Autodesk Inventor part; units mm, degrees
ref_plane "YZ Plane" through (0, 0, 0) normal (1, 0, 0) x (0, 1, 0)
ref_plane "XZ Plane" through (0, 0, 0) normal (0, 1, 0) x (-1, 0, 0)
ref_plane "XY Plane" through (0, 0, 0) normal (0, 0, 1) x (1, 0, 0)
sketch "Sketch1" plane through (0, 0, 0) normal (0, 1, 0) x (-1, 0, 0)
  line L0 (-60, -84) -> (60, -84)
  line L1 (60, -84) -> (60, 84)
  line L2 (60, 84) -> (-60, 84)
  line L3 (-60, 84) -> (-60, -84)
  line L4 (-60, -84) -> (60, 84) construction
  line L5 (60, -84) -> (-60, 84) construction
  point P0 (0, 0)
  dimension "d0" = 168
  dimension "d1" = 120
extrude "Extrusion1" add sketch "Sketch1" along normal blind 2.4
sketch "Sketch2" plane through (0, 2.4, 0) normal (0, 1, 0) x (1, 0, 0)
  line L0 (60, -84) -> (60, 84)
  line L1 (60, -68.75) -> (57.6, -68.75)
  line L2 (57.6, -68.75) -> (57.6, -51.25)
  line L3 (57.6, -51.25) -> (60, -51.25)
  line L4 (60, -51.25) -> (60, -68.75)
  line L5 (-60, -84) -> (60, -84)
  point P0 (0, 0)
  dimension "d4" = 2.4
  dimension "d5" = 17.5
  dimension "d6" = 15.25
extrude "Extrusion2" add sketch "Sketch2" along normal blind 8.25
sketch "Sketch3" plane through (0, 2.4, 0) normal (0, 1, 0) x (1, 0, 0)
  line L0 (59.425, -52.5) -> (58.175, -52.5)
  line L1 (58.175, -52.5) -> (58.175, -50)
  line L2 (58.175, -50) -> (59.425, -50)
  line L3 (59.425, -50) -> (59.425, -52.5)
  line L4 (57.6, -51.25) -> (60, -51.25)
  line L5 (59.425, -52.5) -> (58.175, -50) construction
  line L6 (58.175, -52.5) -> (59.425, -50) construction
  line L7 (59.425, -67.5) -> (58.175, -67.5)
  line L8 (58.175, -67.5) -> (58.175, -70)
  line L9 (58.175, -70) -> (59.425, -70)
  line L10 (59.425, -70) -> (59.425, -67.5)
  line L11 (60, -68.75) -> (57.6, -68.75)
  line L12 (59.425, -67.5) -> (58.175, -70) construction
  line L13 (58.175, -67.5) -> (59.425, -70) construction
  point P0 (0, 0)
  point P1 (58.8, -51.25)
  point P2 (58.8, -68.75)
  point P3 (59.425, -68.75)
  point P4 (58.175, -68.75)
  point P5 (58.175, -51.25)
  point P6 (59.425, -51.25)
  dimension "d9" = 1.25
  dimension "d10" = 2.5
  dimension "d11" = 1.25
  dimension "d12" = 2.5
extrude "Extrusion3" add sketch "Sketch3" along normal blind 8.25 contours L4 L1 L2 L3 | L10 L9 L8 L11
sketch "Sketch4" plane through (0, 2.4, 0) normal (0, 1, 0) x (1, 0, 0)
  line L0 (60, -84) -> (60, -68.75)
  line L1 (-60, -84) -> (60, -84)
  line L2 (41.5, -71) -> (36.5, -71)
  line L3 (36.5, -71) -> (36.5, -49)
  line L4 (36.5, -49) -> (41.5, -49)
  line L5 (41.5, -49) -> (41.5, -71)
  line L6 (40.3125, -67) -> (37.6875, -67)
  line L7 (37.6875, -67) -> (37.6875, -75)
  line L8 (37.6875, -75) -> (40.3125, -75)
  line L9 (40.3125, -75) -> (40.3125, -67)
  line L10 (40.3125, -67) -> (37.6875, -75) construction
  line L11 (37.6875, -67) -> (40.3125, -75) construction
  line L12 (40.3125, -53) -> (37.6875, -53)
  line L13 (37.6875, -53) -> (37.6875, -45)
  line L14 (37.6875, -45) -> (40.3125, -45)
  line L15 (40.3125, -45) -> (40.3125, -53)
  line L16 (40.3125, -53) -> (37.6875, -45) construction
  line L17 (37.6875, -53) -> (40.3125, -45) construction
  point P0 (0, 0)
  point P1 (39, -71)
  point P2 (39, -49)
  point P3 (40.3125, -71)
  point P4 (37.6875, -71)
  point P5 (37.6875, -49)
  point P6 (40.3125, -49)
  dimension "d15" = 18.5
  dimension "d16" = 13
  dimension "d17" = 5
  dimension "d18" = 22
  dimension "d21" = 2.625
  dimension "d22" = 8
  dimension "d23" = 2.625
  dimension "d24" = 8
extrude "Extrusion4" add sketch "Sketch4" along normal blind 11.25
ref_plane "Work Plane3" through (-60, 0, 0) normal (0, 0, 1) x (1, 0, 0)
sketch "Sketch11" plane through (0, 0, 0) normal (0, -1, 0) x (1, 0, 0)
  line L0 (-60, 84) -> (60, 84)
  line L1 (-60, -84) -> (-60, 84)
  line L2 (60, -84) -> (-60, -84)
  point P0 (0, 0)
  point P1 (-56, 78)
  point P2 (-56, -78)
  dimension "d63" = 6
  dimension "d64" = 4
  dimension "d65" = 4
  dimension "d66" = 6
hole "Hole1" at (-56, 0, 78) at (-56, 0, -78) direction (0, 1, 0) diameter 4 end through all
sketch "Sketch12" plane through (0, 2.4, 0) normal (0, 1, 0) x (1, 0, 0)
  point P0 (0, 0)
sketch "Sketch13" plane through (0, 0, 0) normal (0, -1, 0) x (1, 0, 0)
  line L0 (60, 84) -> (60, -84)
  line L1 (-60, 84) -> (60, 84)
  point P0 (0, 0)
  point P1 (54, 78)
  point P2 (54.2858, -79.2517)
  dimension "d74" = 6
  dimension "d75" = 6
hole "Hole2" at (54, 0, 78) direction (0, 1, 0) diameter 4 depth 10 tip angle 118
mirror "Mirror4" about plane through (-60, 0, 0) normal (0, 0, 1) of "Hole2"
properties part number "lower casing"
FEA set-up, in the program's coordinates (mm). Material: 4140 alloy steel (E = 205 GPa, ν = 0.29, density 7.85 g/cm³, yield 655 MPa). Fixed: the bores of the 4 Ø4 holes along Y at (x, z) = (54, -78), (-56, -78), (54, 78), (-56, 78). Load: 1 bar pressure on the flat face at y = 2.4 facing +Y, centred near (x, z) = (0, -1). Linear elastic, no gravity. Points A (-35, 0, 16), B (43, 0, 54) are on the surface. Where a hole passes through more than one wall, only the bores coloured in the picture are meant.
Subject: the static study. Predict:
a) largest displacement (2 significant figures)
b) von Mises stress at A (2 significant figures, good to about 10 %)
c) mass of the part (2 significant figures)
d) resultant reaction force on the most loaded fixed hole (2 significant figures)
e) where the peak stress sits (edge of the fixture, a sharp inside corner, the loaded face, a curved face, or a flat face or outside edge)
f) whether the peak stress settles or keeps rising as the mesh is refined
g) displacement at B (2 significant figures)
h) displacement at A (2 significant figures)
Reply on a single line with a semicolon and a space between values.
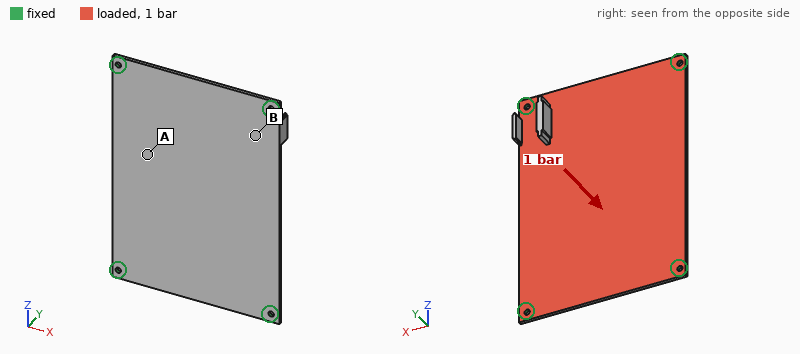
1.2 mm; 120 MPa; 390 g; 520 N; edge of the fixture; keeps rising; 0.40 mm; 1.1 mm
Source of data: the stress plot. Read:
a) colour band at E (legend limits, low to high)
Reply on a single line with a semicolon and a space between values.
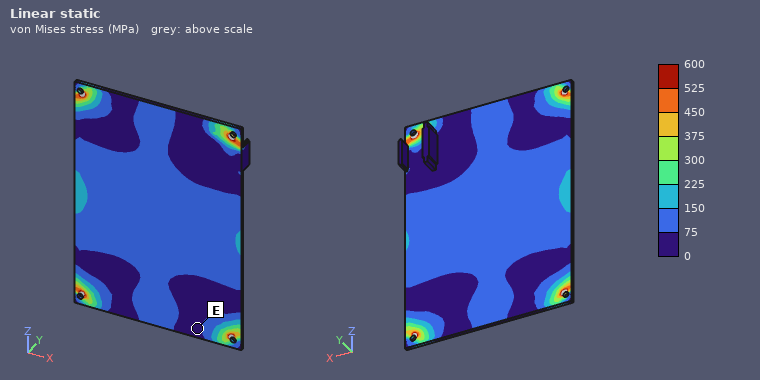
0 to 75 MPa
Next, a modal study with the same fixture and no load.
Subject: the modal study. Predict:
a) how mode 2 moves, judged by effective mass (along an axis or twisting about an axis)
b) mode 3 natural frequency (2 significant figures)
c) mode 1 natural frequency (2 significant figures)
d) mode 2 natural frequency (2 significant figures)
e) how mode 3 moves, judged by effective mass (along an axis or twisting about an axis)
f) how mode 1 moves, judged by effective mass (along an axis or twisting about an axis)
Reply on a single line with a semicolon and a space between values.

twisting about Z; 900 Hz; 380 Hz; 670 Hz; twisting about X; along Y
